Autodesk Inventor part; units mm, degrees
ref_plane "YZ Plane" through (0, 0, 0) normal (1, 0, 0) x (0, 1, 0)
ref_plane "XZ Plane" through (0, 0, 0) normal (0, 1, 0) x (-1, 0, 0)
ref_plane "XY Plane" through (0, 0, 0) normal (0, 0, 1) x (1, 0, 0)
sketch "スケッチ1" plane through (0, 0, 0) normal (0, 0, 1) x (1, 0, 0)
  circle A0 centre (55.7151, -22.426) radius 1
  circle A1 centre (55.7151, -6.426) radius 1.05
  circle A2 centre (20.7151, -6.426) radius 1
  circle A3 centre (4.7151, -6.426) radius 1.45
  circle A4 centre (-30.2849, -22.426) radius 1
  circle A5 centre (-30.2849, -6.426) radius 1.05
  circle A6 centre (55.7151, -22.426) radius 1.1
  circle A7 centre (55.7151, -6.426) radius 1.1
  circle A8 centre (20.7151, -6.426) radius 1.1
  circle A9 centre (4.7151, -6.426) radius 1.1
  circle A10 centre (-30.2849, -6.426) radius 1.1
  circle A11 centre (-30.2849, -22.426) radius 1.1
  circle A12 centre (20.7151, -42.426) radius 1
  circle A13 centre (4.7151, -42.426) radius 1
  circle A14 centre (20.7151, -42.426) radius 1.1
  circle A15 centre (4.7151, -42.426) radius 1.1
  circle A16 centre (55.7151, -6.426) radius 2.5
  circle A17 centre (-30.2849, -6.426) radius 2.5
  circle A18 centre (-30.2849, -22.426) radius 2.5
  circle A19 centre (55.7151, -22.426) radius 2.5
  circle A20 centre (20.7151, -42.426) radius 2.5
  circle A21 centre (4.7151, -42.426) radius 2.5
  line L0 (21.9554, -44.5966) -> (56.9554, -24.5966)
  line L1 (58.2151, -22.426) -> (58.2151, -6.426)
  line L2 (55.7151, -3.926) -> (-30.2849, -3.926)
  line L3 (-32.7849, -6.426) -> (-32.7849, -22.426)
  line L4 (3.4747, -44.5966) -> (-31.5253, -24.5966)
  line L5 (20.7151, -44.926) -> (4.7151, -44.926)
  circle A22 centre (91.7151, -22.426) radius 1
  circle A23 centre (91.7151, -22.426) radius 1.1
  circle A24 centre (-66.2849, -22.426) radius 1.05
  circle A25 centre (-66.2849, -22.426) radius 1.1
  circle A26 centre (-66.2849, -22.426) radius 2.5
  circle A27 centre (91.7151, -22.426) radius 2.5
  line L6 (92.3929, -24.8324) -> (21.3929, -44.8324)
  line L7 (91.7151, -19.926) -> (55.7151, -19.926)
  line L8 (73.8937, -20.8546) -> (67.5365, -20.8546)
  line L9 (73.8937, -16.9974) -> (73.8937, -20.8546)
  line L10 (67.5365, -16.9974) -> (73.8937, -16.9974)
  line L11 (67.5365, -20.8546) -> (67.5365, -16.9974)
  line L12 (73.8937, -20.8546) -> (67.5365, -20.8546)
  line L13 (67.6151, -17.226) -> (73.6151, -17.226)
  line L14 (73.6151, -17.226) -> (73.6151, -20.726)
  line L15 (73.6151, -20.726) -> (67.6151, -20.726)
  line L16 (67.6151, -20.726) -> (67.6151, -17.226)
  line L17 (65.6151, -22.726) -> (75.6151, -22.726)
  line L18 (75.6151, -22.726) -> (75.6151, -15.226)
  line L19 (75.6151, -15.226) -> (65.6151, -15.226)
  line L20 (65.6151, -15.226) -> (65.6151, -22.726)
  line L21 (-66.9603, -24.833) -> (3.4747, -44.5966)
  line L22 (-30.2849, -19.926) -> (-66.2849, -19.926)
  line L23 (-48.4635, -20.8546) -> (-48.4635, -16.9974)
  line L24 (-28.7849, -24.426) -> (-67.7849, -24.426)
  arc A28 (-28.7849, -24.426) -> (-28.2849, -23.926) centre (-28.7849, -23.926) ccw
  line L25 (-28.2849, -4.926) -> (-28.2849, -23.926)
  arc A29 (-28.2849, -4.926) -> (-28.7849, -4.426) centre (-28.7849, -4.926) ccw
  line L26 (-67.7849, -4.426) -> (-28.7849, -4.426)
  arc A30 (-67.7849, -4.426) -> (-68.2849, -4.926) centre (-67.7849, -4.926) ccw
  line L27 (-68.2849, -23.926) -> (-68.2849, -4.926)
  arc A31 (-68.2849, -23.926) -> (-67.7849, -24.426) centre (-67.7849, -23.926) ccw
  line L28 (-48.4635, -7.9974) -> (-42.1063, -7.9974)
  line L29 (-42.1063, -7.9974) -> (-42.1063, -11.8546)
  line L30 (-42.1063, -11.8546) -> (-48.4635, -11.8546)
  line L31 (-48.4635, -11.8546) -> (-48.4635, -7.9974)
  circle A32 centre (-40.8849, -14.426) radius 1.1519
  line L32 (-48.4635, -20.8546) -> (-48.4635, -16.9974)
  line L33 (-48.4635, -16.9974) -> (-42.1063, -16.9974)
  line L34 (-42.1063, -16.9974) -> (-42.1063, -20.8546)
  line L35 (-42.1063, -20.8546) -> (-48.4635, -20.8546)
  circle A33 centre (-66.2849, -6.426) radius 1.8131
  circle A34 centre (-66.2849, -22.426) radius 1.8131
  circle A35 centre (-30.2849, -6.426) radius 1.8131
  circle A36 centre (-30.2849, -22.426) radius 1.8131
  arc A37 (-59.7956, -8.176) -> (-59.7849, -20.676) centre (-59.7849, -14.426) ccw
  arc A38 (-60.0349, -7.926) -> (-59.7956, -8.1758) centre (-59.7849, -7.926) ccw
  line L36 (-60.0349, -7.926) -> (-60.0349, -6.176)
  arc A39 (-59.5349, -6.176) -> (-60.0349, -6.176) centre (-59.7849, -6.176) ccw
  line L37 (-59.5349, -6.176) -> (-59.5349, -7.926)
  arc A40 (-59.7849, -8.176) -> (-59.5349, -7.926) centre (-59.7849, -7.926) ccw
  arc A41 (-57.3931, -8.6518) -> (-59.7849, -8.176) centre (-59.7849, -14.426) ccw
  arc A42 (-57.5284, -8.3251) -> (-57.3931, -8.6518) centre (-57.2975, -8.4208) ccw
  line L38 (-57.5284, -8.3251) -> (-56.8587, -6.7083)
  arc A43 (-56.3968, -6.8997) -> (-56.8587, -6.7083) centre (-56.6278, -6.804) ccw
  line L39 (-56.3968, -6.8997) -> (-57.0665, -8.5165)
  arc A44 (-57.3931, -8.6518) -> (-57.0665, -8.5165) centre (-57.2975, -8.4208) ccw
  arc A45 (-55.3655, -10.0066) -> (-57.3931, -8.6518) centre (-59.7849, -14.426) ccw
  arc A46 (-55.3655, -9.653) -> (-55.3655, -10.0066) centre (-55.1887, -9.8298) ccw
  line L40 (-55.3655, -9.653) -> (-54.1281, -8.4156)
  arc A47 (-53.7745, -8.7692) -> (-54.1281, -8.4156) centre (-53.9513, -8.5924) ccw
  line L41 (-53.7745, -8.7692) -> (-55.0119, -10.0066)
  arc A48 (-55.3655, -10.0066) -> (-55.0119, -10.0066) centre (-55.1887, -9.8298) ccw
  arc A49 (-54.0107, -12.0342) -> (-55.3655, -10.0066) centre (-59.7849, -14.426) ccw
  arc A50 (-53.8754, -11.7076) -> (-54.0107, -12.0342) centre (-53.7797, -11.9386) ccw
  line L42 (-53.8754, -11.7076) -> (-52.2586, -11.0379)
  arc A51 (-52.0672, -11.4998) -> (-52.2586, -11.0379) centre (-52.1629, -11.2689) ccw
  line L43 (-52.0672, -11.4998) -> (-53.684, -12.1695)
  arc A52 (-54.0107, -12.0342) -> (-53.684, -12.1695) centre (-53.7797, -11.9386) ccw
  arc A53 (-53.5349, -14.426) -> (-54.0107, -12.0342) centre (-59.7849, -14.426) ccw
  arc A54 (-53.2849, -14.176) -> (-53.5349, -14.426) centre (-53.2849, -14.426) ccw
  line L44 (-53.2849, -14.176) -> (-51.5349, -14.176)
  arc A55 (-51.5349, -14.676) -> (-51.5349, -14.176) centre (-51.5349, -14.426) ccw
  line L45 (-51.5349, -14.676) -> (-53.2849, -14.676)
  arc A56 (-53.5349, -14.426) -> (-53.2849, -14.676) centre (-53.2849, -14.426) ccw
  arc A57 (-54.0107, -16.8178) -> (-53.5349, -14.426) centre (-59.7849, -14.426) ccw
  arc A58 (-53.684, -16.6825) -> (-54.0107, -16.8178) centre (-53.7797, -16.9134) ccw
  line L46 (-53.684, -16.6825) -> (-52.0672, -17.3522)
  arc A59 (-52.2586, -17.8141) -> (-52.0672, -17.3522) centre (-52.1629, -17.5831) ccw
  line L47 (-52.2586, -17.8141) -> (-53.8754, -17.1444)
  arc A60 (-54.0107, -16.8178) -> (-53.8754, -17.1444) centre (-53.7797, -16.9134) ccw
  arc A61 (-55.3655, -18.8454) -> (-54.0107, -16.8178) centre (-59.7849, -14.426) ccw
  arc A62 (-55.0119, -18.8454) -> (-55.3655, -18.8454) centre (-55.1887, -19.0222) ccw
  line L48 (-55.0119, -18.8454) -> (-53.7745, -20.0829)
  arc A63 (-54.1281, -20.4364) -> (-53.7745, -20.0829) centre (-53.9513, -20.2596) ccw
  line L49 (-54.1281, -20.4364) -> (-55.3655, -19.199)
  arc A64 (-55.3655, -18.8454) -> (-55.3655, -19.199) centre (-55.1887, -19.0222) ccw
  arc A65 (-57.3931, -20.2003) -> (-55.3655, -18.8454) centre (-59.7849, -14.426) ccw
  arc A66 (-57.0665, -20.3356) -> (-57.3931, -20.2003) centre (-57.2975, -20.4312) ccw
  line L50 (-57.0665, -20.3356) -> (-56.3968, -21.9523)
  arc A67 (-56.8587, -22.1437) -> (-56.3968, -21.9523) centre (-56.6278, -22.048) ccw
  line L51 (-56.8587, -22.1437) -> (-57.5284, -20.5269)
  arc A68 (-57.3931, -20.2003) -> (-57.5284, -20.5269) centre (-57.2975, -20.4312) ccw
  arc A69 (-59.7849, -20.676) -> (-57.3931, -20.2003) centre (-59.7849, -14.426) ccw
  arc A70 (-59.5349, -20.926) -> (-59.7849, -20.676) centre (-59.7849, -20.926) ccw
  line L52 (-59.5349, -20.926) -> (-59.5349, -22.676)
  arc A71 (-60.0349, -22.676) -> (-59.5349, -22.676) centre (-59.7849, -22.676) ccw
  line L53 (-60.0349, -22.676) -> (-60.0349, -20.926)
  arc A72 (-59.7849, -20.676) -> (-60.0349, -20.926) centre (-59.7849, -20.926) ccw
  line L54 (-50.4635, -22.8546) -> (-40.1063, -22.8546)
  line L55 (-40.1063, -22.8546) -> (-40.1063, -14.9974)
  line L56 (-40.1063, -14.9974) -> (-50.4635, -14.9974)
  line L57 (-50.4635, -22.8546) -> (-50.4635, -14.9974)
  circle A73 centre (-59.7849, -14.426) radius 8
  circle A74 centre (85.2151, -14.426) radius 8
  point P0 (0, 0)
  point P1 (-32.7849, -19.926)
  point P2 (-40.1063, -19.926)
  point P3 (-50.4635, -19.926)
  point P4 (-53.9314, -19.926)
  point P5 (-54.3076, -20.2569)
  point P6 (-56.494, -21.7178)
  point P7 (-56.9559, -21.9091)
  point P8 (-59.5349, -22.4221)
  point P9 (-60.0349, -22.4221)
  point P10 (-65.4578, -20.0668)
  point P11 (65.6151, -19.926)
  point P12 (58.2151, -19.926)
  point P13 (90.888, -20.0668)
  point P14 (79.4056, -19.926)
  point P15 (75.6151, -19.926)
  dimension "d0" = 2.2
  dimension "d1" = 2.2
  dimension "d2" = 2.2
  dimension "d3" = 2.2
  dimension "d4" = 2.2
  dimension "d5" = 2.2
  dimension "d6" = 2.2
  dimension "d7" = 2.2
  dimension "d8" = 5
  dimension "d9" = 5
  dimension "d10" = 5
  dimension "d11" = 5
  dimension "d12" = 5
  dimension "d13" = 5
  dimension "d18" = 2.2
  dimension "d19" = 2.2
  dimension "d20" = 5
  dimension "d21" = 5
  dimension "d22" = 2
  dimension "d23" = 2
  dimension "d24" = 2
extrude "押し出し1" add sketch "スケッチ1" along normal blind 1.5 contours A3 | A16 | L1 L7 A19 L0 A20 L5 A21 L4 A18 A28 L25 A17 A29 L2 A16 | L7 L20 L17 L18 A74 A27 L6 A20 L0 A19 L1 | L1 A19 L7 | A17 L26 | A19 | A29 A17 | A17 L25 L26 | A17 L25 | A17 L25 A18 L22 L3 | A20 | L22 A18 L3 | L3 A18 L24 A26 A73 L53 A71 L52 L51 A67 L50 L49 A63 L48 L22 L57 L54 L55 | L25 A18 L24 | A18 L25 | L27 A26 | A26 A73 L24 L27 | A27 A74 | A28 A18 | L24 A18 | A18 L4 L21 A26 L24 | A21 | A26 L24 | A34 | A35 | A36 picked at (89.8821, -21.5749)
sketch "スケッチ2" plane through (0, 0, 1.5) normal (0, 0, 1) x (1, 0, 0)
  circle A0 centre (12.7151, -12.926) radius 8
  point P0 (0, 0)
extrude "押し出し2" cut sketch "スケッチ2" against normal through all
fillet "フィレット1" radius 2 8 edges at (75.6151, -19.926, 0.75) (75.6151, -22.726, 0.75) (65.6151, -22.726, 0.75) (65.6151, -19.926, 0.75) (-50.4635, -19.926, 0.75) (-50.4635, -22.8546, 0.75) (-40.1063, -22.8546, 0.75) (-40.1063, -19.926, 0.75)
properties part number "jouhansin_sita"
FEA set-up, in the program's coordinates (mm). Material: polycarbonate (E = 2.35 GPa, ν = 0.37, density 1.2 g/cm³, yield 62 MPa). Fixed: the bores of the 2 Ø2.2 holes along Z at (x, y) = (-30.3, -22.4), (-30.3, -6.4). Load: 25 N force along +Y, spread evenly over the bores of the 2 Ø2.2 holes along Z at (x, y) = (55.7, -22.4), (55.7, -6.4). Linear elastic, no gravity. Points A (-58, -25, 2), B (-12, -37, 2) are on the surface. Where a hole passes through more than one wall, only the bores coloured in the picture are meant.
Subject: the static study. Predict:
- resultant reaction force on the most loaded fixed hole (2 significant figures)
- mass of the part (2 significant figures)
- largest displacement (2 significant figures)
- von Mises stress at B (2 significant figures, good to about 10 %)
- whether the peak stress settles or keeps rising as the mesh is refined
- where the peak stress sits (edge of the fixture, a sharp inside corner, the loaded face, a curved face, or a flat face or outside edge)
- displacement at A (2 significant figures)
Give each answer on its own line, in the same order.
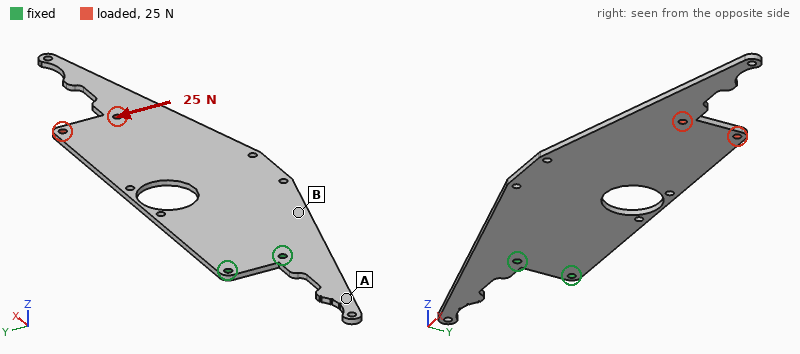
130 N
6.6 g
1.5 mm
4.0 MPa
keeps rising
edge of the fixture
0.26 mm
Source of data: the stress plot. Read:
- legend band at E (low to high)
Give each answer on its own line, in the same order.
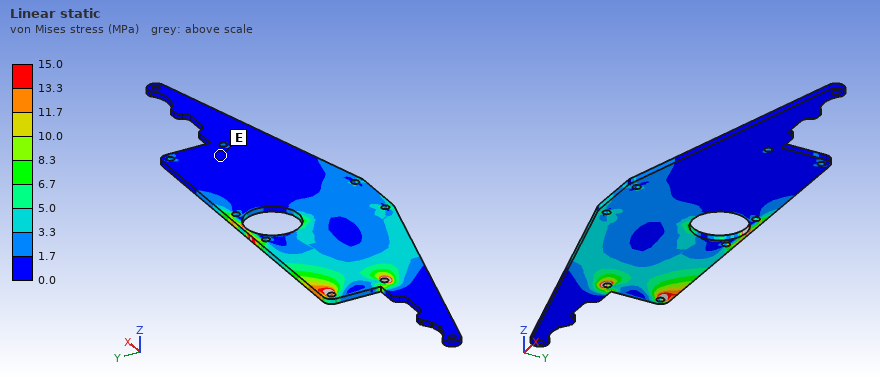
0.0 to 1.7 MPa
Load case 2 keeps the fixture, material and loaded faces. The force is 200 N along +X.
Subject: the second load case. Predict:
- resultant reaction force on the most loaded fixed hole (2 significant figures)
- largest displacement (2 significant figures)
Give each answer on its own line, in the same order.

100 N
1.5 mm
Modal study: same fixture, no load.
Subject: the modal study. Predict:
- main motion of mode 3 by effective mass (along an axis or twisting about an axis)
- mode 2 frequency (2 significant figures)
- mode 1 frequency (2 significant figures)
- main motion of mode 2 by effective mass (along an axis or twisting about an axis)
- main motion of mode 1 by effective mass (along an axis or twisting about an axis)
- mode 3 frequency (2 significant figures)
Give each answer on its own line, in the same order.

twisting about X
170 Hz
33 Hz
along Z
along Z
190 Hz
